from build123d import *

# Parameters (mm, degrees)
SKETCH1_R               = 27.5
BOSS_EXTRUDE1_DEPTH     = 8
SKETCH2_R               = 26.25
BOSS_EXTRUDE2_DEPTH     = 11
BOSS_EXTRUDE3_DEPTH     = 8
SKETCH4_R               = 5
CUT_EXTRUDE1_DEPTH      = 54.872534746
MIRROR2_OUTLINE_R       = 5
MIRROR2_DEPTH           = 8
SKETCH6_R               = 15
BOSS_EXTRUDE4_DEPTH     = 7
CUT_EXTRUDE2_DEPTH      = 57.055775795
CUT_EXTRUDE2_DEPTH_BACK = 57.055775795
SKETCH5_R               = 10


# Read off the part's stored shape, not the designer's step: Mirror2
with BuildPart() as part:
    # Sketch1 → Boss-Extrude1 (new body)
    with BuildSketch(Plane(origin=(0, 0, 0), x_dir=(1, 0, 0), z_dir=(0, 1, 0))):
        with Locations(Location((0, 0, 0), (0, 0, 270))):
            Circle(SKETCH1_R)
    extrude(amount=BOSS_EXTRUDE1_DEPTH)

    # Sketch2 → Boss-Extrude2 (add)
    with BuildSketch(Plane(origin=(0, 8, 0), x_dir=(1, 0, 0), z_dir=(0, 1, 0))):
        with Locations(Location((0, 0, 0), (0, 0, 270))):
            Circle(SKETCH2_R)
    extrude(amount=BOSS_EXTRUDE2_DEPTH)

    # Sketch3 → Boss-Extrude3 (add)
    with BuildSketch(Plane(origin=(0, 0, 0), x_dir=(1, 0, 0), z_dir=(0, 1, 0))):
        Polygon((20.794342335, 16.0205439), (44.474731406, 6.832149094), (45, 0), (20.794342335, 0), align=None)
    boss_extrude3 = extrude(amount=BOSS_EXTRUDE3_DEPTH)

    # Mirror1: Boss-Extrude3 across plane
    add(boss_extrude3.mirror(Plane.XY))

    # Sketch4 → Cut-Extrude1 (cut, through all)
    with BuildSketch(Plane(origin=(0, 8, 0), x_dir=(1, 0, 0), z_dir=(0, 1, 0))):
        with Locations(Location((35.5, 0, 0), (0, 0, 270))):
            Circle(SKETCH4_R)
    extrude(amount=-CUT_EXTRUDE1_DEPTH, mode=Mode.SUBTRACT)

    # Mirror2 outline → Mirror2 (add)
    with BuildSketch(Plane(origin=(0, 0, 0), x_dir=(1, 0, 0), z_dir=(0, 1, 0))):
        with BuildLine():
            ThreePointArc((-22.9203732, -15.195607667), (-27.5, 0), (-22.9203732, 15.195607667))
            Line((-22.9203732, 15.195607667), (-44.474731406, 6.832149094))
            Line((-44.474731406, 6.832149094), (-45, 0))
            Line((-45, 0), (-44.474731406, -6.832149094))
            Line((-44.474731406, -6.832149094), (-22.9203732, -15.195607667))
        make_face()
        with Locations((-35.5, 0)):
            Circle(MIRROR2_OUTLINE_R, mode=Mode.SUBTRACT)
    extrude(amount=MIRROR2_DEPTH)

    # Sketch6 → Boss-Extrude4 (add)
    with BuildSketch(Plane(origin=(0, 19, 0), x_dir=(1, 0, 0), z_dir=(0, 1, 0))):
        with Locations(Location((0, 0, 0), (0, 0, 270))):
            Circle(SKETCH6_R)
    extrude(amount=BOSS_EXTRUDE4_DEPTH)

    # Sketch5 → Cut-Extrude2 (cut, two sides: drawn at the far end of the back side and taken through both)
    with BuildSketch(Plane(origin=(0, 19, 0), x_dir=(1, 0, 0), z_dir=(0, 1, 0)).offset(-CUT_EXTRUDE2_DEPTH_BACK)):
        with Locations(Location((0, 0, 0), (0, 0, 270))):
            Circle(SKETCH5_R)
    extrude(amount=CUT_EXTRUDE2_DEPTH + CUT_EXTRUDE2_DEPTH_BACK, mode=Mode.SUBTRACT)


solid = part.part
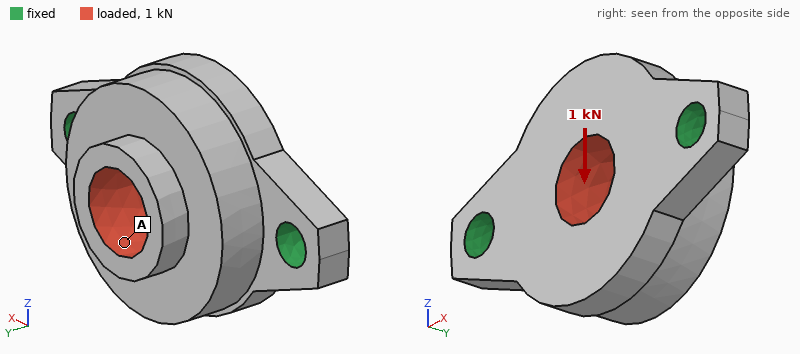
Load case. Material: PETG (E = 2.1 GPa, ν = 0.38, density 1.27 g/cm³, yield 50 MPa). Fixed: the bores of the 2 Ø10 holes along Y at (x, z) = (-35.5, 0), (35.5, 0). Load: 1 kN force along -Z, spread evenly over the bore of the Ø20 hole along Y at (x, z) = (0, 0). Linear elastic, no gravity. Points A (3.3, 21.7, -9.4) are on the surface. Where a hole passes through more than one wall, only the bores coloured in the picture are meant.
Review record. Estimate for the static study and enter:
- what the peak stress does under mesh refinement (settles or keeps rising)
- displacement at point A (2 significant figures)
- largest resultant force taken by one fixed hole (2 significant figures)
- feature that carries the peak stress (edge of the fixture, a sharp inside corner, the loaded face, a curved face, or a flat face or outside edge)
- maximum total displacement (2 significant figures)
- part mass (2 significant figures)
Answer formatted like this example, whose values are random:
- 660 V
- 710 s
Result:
- keeps rising
- 0.31 mm
- 500 N
- edge of the fixture
- 0.41 mm
- 56 g
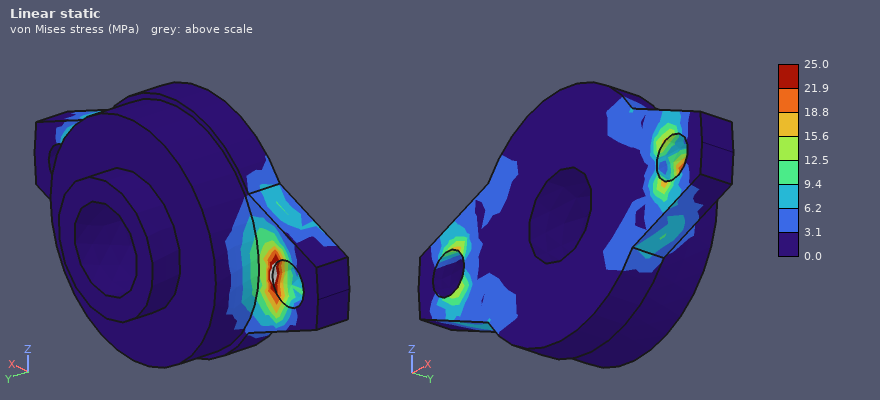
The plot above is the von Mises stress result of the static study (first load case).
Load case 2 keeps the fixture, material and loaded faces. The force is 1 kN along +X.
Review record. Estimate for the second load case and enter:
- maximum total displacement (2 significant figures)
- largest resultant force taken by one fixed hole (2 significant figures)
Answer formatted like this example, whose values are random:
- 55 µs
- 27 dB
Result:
- 48 µm
- 520 N
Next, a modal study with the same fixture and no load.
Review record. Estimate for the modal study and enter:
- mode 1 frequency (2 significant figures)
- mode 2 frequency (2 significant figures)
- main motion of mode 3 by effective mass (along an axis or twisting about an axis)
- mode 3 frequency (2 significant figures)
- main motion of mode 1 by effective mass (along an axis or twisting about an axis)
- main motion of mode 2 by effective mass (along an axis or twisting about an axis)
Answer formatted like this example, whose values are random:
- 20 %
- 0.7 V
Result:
- 1100 Hz
- 2100 Hz
- along Z
- 3300 Hz
- along Z
- along Y
